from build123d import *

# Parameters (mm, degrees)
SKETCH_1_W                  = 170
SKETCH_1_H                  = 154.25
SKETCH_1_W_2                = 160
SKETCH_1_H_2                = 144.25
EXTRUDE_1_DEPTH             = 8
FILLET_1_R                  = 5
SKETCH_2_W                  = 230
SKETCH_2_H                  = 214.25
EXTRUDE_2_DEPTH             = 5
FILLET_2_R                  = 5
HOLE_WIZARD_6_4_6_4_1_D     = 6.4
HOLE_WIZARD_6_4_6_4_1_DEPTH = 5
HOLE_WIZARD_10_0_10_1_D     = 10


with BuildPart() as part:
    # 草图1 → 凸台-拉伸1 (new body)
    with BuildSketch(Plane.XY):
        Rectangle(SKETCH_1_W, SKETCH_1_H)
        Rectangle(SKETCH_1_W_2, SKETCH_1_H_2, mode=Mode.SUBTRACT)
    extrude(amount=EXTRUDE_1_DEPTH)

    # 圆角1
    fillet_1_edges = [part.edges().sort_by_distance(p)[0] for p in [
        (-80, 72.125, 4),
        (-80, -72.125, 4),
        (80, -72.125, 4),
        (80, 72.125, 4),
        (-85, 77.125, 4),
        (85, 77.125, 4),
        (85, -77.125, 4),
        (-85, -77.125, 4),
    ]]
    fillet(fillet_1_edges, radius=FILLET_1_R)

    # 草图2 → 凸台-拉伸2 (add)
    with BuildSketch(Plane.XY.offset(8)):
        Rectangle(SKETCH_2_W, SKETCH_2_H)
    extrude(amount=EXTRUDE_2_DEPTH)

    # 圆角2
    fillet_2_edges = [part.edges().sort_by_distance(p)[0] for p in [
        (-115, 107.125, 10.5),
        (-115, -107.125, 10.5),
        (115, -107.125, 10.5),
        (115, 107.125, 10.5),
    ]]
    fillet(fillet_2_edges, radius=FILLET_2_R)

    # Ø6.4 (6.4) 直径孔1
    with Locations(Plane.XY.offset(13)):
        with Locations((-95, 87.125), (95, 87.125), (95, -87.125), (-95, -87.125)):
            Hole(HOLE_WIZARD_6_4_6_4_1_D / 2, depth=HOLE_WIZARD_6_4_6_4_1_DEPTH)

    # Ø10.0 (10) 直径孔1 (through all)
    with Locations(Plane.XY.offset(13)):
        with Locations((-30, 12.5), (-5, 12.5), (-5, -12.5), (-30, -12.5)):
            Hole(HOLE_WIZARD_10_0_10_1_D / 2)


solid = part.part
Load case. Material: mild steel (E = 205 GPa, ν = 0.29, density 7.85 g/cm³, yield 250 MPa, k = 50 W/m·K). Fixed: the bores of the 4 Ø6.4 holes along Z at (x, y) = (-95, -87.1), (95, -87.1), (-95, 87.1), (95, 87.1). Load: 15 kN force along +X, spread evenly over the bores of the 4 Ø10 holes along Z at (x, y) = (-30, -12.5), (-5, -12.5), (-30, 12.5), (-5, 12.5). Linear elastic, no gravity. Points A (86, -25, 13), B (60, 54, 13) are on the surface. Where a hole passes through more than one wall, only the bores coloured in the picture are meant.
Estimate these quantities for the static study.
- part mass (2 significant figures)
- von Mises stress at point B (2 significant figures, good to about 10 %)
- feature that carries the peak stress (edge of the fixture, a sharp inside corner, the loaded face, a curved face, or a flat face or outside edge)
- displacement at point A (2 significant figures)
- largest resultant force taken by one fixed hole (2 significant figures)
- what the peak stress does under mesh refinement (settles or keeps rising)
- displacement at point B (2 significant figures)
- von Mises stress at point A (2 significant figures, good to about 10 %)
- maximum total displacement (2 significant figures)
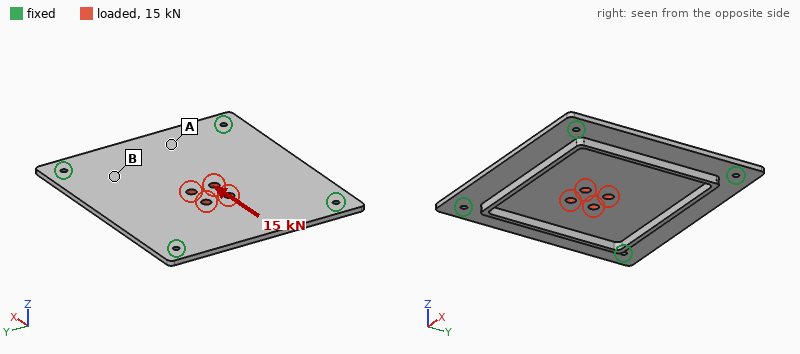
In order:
2.1 kg
14 MPa
edge of the fixture
7.1 µm
4.2 kN
keeps rising
5.6 µm
5.3 MPa
14 µm
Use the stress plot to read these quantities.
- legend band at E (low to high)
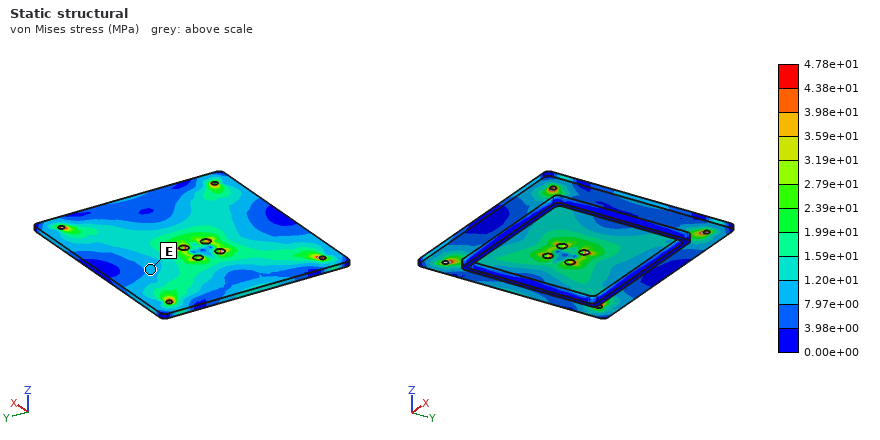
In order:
7.97e+00 to 1.20e+01 MPa
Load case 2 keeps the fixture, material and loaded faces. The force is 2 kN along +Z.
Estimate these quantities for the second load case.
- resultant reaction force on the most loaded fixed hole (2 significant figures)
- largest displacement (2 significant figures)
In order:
1.0 kN
0.32 mm
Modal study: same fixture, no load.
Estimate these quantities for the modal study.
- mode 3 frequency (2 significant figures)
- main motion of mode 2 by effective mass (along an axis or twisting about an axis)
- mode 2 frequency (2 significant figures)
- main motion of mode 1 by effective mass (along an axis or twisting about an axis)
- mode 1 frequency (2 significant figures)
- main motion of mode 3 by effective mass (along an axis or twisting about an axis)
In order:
1100 Hz
twisting about X
970 Hz
along Z
610 Hz
twisting about Y
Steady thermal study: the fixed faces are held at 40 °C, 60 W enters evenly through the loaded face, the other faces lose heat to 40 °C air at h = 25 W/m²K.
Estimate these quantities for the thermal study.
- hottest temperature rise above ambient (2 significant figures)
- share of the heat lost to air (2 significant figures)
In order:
70 K
74 %
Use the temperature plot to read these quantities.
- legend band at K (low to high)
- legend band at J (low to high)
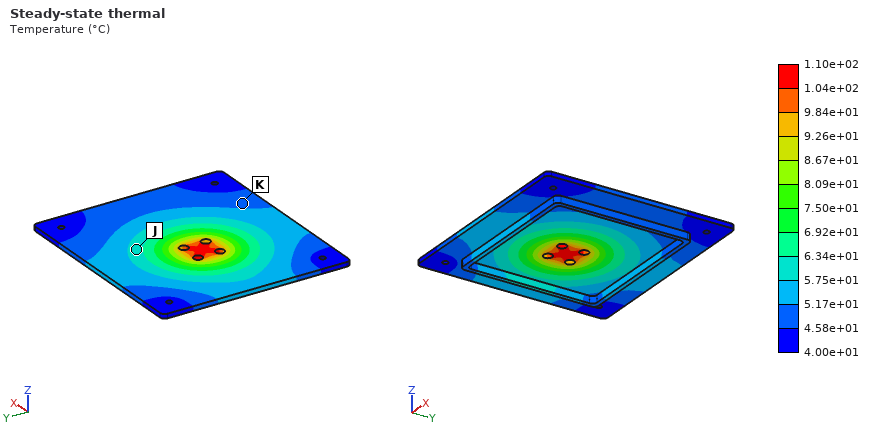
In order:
4.58e+01 to 5.17e+01 °C
5.75e+01 to 6.34e+01 °C
